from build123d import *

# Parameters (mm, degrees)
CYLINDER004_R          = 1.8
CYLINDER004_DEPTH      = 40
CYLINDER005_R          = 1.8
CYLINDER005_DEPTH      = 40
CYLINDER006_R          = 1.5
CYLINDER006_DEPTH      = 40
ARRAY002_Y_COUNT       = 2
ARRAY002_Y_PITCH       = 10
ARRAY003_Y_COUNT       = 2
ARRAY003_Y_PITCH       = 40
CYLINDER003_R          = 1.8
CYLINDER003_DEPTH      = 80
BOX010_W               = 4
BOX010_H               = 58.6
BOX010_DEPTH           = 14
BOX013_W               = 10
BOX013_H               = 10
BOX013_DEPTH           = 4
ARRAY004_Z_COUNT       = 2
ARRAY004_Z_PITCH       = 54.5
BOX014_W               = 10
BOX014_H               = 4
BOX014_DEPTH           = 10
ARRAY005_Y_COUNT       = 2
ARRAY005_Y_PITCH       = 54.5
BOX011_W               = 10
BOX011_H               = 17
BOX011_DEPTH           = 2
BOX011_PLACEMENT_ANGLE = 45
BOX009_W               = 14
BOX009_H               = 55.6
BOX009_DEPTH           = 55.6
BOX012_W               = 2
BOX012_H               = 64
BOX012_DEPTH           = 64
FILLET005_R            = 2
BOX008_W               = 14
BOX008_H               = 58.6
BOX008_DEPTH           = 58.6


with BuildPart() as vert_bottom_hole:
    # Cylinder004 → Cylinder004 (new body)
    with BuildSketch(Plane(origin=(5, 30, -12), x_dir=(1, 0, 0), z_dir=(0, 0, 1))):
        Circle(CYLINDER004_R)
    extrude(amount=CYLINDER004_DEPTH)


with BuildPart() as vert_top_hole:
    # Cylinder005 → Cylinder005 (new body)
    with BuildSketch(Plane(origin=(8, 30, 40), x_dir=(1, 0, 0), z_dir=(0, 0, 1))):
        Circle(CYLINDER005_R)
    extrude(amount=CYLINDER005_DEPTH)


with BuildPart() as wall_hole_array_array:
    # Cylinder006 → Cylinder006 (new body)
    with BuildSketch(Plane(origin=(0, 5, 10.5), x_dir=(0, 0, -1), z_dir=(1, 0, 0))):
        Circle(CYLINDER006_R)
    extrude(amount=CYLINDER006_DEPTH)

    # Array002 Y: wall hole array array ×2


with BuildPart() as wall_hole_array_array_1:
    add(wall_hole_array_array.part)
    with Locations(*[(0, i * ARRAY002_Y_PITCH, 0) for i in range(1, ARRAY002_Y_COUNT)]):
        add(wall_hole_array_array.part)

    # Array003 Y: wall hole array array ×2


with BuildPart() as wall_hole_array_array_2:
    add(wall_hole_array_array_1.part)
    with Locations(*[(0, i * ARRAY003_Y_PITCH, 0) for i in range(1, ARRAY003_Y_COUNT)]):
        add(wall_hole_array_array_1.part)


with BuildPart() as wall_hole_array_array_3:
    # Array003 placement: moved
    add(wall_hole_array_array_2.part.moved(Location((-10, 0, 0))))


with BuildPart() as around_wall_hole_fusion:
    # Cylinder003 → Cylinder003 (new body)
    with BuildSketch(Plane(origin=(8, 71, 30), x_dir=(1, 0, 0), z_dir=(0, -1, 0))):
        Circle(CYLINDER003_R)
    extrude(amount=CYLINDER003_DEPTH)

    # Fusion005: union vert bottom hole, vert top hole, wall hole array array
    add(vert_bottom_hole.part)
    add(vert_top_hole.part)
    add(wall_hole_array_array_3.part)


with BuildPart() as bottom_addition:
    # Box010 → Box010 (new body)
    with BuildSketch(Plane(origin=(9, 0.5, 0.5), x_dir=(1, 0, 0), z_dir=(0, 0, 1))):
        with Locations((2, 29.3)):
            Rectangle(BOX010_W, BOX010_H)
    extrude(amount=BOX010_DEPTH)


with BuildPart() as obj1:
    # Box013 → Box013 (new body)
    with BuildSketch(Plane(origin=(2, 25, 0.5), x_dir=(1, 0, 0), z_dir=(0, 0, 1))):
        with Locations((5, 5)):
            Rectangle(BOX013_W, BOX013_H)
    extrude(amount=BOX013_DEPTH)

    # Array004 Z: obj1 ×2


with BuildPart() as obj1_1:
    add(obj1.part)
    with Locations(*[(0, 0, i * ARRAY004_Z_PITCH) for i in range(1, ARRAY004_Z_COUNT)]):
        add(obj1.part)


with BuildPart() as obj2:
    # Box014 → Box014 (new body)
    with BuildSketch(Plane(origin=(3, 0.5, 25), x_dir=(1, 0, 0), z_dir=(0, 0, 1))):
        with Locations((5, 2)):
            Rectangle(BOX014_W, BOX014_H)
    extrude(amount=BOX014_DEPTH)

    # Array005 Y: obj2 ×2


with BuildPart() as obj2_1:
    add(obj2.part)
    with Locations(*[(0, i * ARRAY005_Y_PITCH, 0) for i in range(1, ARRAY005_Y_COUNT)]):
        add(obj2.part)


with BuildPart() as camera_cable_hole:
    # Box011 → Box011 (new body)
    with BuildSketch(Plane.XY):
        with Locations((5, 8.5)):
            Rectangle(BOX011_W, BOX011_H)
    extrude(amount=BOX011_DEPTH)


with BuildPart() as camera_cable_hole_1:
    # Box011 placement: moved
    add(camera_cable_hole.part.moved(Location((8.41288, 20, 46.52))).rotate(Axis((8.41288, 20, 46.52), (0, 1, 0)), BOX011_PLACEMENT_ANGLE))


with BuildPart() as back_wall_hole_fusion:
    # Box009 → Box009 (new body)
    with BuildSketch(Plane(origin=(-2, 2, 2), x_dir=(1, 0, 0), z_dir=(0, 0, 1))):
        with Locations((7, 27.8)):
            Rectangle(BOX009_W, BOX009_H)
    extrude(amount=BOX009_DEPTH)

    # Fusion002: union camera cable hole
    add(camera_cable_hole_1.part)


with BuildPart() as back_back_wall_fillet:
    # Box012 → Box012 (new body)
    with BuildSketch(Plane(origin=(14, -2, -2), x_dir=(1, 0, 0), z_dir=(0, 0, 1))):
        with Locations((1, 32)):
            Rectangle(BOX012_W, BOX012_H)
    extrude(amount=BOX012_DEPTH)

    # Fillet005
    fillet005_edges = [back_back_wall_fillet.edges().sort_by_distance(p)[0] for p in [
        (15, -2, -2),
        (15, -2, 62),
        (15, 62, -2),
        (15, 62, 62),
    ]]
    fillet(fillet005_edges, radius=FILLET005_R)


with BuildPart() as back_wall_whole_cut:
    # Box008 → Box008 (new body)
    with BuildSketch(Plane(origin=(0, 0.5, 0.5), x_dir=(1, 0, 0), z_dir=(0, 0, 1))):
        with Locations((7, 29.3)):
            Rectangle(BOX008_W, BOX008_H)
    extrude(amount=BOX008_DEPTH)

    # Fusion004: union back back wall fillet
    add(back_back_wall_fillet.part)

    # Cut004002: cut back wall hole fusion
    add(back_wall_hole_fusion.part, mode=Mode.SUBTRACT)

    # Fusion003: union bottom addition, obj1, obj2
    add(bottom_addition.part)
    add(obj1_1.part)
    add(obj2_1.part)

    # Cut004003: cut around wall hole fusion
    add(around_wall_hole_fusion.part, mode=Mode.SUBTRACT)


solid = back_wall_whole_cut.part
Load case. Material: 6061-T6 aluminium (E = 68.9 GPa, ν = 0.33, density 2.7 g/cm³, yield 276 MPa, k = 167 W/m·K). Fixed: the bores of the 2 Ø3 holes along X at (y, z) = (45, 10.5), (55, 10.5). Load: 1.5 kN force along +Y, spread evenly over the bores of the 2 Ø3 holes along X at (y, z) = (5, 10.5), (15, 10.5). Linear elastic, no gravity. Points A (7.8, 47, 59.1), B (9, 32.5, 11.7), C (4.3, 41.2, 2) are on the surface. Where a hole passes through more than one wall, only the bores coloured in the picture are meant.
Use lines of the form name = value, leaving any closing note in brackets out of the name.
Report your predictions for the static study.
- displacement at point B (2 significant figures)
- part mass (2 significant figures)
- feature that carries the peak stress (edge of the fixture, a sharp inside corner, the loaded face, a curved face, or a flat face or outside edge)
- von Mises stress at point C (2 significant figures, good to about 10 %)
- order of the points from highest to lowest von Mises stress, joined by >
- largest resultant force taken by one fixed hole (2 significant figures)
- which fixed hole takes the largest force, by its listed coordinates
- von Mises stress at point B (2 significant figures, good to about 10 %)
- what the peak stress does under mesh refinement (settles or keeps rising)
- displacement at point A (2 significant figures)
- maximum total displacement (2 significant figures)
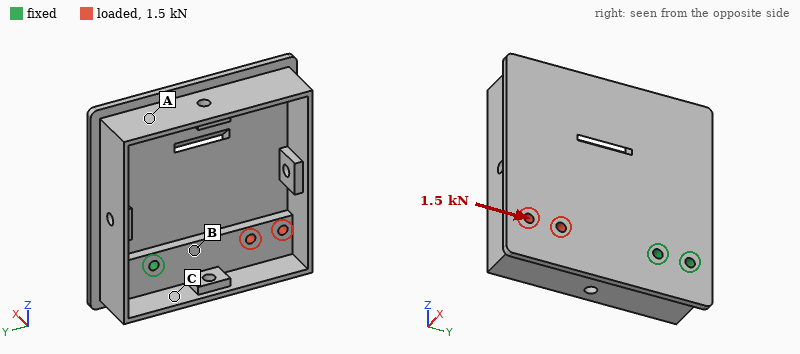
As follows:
displacement at point B = 2.6 µm
part mass = 58 g
feature that carries the peak stress = edge of the fixture
von Mises stress at point C = 5.1 MPa
order of the points from highest to lowest von Mises stress, joined by > = B > C > A
largest resultant force taken by one fixed hole = 1.1 kN
which fixed hole takes the largest force, by its listed coordinates = (45, 10.5)
von Mises stress at point B = 12 MPa
what the peak stress does under mesh refinement = keeps rising
displacement at point A = 3.8 µm
maximum total displacement = 7.7 µm
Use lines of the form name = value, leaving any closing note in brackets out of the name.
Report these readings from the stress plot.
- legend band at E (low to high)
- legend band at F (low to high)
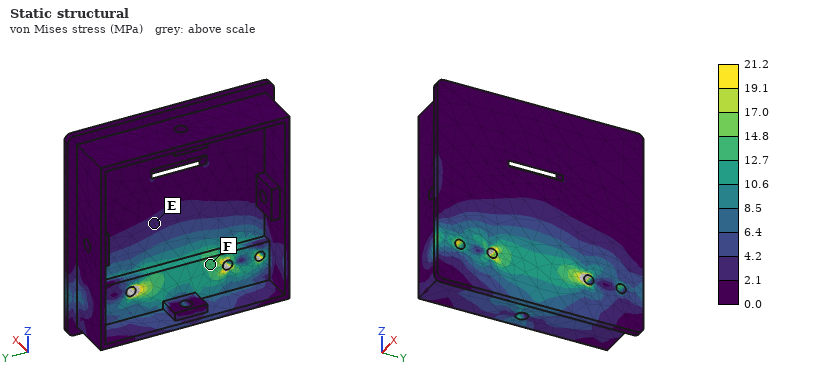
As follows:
legend band at E = 2.1 to 4.2 MPa
legend band at F = 12.7 to 14.8 MPa
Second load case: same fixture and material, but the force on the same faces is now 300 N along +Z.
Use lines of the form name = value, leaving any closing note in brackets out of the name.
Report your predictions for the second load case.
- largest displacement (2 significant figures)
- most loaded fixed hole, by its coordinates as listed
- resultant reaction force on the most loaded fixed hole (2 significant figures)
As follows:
largest displacement = 34 µm
most loaded fixed hole, by its coordinates as listed = (45, 10.5)
resultant reaction force on the most loaded fixed hole = 1.1 kN
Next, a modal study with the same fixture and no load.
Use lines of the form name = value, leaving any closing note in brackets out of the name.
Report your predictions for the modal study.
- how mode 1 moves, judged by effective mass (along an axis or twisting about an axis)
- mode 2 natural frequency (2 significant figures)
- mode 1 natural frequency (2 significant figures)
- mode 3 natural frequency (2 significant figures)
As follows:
how mode 1 moves, judged by effective mass = along X
mode 2 natural frequency = 2400 Hz
mode 1 natural frequency = 1200 Hz
mode 3 natural frequency = 3100 Hz
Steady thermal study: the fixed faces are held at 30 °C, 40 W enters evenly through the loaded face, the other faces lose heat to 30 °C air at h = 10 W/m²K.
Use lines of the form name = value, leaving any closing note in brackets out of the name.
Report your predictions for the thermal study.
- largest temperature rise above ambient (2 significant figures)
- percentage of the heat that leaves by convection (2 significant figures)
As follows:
largest temperature rise above ambient = 47 K
percentage of the heat that leaves by convection = 7.8 %
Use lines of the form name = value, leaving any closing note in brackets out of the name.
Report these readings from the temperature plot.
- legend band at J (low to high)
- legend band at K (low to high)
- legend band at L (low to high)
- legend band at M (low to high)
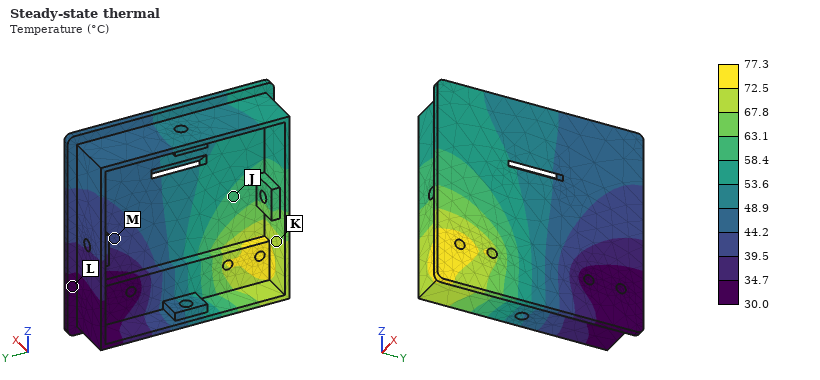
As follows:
legend band at J = 58.4 to 63.1 °C
legend band at K = 67.8 to 72.5 °C
legend band at L = 30.0 to 34.7 °C
legend band at M = 39.5 to 44.2 °C
